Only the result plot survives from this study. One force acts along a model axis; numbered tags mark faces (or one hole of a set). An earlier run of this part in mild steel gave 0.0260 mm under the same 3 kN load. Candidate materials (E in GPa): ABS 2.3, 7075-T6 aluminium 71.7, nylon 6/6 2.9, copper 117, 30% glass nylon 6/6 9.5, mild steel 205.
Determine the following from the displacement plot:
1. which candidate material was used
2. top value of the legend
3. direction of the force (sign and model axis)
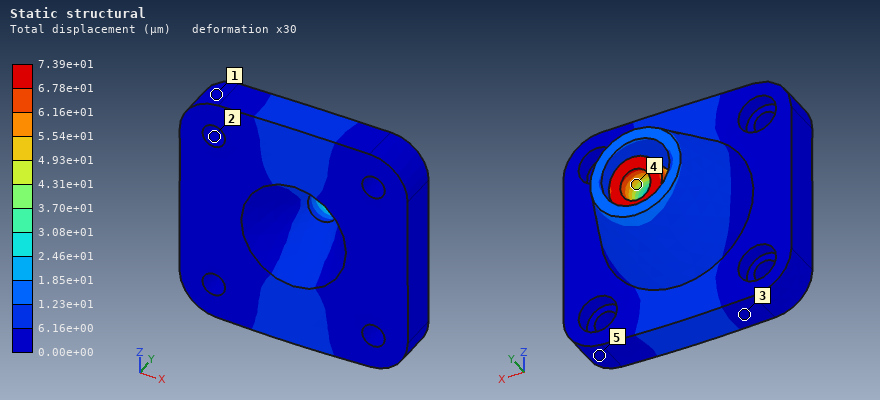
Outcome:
7075-T6 aluminium
7.39e+01 µm
-Z
